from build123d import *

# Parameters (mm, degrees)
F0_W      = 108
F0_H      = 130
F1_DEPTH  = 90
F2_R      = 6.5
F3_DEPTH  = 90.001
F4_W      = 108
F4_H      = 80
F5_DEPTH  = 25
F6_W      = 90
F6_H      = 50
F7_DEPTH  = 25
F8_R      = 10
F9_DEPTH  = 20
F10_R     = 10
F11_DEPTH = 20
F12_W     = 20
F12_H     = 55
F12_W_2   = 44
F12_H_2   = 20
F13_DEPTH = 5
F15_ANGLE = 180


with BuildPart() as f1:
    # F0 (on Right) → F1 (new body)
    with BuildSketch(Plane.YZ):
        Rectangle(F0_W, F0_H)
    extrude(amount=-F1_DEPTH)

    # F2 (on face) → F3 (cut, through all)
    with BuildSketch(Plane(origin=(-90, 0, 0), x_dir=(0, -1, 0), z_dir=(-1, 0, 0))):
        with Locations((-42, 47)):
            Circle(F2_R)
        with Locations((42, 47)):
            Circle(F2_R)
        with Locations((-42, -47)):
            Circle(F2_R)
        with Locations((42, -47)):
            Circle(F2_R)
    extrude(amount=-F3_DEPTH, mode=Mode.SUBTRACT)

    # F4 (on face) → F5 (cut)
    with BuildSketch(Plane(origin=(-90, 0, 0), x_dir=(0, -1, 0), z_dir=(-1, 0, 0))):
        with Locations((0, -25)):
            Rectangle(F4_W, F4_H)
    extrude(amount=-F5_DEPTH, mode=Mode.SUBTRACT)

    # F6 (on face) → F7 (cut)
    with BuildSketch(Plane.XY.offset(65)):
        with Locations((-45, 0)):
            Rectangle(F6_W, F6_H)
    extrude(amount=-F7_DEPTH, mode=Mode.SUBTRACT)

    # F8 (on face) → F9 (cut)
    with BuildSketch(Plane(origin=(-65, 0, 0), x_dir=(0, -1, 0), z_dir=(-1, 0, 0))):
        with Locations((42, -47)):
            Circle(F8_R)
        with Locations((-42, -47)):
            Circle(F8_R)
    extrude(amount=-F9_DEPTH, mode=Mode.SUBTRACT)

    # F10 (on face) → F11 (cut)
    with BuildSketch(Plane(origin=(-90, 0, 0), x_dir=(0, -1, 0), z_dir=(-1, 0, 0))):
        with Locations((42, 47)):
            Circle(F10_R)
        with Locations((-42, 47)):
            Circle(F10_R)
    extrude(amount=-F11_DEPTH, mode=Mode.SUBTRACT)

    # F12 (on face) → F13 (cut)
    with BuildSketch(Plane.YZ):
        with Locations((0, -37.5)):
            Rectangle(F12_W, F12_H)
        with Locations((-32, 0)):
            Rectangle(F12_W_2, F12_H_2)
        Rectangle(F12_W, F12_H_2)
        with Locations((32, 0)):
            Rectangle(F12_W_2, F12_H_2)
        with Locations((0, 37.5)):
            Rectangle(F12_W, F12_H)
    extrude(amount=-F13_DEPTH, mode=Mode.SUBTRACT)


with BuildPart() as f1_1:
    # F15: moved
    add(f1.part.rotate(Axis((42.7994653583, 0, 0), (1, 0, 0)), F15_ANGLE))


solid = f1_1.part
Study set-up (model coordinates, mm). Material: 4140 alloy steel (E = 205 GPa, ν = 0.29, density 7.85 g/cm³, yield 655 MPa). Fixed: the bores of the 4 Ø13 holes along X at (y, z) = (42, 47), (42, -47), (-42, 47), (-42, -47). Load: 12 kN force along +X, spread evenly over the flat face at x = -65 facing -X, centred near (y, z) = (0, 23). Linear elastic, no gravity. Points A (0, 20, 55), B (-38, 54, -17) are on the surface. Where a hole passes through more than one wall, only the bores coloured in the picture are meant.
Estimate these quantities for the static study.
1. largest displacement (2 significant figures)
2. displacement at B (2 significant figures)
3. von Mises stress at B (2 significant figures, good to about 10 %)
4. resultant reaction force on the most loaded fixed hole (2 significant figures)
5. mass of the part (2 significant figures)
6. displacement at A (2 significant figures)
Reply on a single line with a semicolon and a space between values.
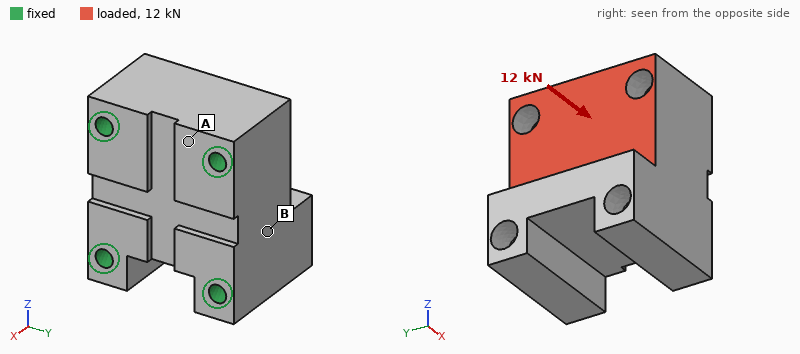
0.70 µm; 0.32 µm; 1.6 MPa; 4.2 kN; 6.8 kg; 0.33 µm
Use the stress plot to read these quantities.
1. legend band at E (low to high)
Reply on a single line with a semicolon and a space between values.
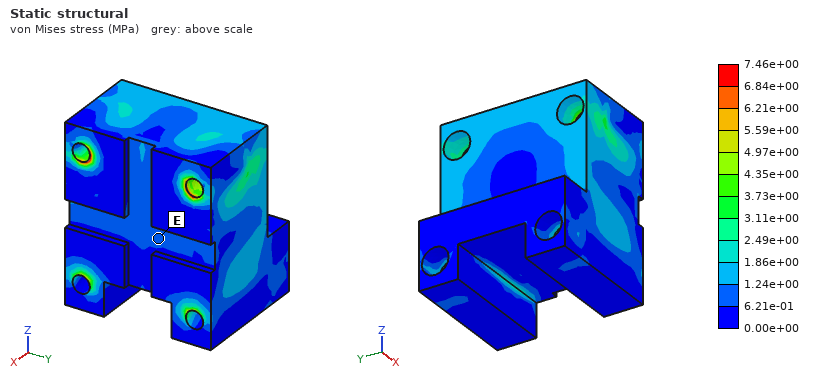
6.21e-01 to 1.24e+00 MPa
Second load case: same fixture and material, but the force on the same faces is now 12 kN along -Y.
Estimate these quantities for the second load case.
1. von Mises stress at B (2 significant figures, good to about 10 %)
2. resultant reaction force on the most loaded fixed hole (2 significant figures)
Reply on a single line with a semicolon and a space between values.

2.1 MPa; 4.9 kN
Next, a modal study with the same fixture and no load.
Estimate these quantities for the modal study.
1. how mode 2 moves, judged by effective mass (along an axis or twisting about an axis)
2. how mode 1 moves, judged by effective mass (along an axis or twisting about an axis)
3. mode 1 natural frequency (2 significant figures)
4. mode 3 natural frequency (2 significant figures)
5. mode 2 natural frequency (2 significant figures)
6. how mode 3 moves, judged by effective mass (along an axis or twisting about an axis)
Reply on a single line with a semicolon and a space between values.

along Y; along X; 11 kHz; 14 kHz; 12 kHz; along Z
